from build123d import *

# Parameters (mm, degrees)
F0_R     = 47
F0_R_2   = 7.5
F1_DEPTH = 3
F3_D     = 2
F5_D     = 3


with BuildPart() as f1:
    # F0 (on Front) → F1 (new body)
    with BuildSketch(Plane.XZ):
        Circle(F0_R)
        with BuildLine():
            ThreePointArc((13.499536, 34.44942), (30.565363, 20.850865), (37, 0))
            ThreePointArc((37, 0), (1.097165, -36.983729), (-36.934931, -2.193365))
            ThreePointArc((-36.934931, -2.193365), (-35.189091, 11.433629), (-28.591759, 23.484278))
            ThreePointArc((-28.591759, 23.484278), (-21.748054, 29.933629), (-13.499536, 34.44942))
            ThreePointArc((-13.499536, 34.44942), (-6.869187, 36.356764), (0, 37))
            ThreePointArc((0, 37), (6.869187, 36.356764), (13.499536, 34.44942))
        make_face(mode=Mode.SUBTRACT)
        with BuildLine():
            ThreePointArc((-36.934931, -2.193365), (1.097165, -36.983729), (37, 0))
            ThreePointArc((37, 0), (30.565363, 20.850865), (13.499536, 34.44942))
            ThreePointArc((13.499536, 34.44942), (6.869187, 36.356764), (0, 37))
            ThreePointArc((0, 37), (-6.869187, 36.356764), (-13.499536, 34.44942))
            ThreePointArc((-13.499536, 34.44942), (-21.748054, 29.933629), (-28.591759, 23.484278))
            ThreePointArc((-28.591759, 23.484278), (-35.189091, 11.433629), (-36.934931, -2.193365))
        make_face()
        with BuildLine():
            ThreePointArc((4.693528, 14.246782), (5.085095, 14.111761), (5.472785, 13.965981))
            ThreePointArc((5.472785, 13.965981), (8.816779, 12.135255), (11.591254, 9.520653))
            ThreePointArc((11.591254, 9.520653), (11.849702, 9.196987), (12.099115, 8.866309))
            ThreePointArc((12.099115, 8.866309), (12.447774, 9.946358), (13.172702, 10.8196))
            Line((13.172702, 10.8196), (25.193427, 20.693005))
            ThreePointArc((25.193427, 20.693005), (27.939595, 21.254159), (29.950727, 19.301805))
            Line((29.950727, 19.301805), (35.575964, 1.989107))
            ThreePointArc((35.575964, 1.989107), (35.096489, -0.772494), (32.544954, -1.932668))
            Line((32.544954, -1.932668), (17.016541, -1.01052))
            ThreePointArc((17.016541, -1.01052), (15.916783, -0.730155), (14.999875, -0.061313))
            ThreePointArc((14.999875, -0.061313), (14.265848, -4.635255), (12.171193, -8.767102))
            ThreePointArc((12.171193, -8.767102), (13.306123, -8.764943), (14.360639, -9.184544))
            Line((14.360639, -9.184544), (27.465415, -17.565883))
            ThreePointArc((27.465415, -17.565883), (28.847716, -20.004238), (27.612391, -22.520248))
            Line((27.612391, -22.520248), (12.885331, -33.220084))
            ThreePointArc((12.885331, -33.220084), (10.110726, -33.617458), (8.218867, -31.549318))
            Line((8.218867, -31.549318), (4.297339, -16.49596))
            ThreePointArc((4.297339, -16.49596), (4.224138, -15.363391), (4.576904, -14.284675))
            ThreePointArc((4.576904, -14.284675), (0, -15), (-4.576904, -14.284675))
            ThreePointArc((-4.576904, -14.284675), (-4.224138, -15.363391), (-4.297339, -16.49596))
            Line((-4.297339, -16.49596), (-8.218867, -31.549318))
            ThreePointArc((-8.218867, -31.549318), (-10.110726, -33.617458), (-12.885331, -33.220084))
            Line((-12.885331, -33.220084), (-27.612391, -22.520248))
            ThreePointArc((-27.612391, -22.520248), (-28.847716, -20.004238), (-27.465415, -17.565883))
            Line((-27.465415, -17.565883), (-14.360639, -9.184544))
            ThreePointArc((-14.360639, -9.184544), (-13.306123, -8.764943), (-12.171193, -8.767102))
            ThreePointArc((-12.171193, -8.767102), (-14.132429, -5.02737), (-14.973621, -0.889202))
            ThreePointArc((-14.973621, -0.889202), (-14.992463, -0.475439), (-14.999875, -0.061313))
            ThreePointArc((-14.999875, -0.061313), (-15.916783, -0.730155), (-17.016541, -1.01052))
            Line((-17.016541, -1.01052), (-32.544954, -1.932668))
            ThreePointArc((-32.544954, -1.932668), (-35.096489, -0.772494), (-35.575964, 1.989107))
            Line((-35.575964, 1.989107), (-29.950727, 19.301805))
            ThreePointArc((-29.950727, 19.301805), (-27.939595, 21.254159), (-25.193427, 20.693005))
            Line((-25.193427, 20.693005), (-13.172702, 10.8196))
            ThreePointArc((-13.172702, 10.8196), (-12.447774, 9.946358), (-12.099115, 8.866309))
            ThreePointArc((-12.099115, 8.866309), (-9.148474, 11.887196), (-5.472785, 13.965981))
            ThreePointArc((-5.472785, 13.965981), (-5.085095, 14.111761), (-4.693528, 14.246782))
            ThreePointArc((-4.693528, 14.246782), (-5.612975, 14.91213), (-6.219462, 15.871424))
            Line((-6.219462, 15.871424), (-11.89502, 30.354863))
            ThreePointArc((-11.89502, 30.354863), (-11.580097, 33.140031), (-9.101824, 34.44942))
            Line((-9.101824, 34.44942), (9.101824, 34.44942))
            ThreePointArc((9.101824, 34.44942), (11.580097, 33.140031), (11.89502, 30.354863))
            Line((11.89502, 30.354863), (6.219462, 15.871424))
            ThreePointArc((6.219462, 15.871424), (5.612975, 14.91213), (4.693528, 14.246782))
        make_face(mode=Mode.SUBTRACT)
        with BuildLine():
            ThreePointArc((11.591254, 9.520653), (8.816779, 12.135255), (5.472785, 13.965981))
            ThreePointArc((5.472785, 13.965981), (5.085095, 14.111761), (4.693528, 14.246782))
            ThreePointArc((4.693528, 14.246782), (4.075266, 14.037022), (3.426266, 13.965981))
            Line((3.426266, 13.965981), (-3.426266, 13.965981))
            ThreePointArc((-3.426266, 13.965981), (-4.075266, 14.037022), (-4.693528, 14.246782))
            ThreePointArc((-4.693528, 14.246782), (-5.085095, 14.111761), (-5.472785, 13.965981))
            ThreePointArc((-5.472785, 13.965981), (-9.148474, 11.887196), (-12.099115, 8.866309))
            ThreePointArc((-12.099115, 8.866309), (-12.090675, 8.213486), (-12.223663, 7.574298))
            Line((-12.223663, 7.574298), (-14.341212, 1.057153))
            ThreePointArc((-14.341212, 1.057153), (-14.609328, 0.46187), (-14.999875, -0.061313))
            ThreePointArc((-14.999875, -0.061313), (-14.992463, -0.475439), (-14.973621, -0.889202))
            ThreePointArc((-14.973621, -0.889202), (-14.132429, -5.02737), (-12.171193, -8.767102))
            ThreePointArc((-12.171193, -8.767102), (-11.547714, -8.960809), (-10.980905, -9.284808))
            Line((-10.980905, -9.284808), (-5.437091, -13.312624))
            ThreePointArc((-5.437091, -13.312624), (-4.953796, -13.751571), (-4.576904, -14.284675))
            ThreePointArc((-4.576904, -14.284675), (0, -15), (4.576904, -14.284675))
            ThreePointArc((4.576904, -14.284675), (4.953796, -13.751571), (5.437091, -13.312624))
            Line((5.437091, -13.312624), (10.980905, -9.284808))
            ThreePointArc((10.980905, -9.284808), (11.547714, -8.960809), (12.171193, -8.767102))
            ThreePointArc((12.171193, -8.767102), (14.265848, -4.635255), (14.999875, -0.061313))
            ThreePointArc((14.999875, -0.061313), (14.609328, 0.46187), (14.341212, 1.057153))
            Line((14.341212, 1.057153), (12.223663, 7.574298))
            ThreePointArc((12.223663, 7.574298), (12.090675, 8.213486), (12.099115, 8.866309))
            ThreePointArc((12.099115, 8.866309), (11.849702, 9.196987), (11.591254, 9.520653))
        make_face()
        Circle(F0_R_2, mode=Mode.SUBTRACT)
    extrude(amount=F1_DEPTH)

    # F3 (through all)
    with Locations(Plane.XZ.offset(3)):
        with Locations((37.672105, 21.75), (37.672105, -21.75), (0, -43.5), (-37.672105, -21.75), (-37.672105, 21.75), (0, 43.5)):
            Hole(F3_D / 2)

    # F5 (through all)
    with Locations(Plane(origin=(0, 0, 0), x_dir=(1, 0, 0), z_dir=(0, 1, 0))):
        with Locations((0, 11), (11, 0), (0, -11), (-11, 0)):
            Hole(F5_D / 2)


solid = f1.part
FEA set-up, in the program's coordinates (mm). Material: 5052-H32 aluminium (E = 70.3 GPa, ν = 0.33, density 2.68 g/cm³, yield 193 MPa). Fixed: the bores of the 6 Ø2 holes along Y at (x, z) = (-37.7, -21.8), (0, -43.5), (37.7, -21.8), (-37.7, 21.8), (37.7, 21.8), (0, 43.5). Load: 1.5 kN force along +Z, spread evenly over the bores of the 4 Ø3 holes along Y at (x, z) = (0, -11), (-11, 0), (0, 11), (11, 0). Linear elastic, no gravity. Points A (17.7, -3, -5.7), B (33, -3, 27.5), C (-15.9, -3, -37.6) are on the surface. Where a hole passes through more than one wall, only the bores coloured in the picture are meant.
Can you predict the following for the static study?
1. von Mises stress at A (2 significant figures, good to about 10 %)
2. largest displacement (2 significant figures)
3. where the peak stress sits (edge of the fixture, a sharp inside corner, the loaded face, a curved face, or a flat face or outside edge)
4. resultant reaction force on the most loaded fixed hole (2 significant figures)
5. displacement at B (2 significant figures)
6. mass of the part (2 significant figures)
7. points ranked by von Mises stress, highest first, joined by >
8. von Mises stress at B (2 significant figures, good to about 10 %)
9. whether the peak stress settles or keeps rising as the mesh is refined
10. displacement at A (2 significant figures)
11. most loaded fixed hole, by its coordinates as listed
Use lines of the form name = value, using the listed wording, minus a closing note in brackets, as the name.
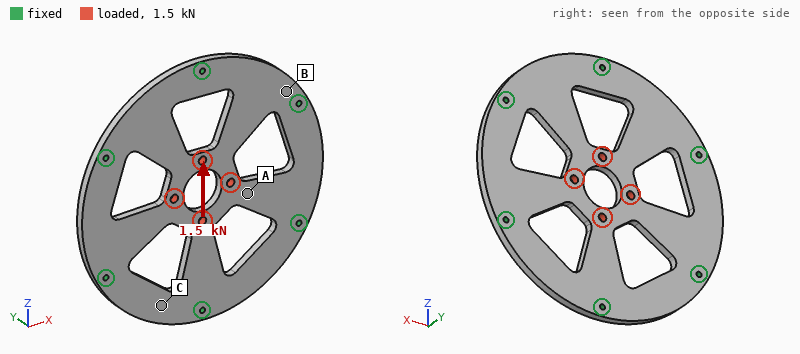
von Mises stress at A = 13 MPa
largest displacement = 13 µm
where the peak stress sits = edge of the fixture
resultant reaction force on the most loaded fixed hole = 530 N
displacement at B = 2.2 µm
mass of the part = 39 g
points ranked by von Mises stress, highest first, joined by > = A > B > C
von Mises stress at B = 6.9 MPa
whether the peak stress settles or keeps rising as the mesh is refined = keeps rising
displacement at A = 6.7 µm
most loaded fixed hole, by its coordinates as listed = (0, -43.5)
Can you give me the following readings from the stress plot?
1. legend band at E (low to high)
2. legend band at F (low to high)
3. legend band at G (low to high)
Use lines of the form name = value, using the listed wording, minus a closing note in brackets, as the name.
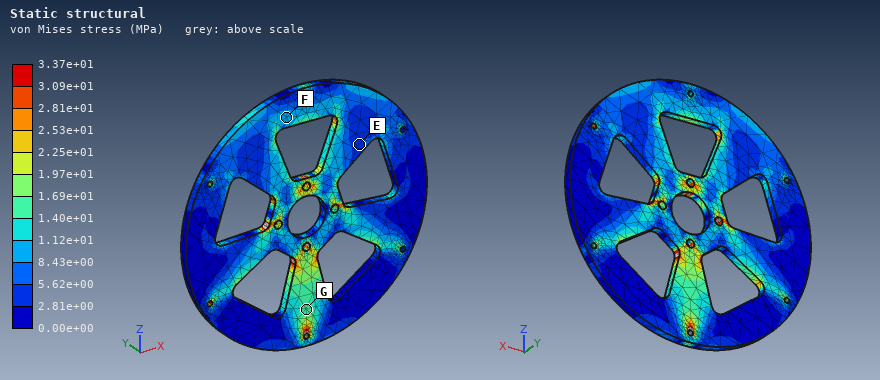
legend band at E = 2.81e+00 to 5.62e+00 MPa
legend band at F = 8.43e+00 to 1.12e+01 MPa
legend band at G = 1.40e+01 to 1.69e+01 MPa
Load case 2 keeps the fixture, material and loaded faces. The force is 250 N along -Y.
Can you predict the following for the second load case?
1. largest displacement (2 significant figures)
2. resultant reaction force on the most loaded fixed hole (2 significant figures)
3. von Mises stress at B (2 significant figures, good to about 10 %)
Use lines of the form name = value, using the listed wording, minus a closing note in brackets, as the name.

largest displacement = 0.15 mm
resultant reaction force on the most loaded fixed hole = 44 N
von Mises stress at B = 20 MPa
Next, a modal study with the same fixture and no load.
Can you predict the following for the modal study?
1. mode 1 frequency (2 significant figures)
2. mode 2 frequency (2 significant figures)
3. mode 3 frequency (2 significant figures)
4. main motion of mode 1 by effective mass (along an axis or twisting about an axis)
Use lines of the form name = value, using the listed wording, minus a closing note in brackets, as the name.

mode 1 frequency = 2800 Hz
mode 2 frequency = 5800 Hz
mode 3 frequency = 5800 Hz
main motion of mode 1 by effective mass = along Y
